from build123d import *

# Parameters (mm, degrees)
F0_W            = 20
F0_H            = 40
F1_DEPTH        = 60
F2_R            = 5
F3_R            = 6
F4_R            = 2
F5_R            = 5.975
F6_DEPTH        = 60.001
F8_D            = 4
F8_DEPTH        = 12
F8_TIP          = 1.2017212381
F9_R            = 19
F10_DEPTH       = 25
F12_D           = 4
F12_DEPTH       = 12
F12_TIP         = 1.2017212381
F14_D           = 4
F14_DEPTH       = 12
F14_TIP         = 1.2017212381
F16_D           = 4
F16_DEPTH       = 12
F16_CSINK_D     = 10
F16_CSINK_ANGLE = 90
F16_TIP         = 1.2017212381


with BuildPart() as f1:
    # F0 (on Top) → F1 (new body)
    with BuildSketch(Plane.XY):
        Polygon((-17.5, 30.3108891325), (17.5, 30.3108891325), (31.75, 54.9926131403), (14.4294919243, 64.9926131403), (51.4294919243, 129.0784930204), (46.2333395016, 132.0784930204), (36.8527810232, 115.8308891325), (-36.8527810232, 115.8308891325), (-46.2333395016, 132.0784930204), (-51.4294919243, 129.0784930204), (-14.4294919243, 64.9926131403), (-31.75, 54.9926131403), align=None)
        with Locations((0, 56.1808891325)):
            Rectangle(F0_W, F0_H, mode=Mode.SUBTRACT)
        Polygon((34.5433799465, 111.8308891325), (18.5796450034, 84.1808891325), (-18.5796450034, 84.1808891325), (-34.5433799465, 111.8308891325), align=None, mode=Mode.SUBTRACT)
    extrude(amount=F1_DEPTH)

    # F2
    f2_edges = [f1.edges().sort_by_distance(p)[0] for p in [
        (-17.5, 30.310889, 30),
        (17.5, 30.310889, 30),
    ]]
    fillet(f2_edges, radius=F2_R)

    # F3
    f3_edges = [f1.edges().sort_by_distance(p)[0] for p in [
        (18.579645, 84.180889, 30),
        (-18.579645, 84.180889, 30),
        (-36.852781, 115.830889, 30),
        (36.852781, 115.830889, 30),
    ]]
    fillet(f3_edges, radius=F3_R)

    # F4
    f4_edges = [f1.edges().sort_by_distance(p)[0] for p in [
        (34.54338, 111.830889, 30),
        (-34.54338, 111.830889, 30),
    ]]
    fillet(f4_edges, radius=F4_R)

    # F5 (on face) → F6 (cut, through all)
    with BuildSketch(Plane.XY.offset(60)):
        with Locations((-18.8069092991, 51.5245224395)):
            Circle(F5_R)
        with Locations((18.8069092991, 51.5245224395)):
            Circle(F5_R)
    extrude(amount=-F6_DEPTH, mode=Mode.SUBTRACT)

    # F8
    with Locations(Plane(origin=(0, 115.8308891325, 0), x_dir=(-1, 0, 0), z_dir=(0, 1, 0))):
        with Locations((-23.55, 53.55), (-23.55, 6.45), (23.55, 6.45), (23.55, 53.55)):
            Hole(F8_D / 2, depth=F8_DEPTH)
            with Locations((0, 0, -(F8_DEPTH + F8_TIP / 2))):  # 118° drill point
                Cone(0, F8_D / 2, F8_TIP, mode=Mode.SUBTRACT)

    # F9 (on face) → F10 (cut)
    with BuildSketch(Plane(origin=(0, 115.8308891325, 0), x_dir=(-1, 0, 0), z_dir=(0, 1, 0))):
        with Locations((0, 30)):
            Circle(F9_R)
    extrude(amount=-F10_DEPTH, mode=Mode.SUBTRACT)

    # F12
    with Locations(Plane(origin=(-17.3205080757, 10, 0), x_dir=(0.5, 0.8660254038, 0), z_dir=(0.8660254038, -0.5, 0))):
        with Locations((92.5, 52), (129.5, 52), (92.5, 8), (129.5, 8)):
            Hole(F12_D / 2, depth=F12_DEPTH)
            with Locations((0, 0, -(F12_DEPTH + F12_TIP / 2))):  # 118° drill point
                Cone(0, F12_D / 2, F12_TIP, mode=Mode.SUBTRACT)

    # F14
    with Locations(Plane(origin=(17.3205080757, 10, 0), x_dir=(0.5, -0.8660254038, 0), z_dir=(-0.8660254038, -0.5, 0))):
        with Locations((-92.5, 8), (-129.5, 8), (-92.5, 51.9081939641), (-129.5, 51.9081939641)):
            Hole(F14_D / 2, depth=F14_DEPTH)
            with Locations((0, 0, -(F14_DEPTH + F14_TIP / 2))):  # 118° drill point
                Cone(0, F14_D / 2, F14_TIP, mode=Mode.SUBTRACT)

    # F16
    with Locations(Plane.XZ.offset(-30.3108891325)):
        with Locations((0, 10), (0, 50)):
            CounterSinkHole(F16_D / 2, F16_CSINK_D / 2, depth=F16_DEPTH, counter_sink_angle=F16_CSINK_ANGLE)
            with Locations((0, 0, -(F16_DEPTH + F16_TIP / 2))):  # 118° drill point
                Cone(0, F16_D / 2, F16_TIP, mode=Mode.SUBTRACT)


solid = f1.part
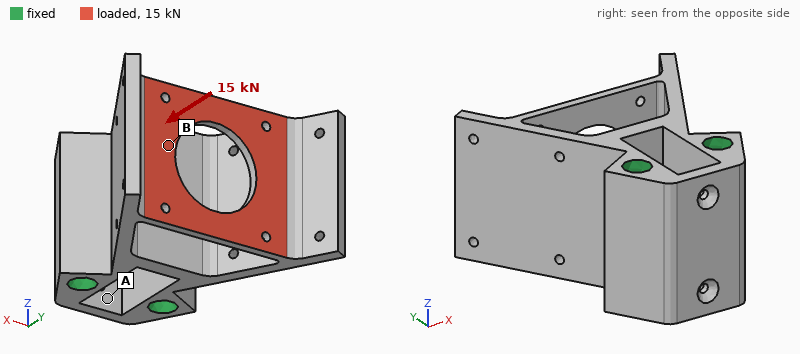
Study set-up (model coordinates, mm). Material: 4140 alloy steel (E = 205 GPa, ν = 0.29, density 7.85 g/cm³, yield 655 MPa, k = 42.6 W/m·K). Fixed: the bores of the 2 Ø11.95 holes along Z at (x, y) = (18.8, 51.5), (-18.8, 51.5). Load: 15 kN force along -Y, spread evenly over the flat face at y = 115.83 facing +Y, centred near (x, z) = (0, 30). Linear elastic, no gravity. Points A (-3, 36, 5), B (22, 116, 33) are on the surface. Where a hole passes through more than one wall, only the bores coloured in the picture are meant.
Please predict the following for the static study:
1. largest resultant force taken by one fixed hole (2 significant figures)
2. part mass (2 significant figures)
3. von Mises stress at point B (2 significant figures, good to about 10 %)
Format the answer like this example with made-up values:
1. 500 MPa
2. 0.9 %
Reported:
1. 9.0 kN
2. 1.1 kg
3. 100 MPa
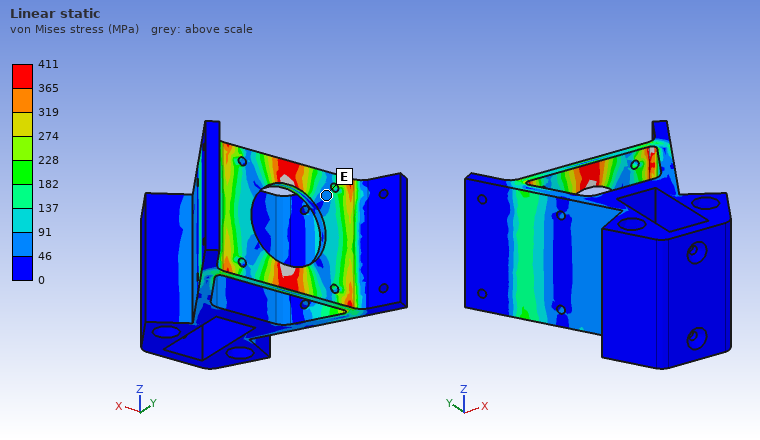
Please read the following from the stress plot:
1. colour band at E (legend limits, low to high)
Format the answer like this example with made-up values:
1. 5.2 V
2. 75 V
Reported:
1. 46 to 91 MPa
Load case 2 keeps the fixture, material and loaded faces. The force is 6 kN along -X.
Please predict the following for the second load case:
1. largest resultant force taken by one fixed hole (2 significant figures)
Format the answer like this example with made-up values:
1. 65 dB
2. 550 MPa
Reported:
1. 10 kN
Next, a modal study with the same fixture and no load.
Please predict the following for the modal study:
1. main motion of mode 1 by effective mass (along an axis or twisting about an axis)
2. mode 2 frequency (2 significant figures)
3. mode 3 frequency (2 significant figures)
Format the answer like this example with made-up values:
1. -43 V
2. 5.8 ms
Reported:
1. along X
2. 4000 Hz
3. 4200 Hz
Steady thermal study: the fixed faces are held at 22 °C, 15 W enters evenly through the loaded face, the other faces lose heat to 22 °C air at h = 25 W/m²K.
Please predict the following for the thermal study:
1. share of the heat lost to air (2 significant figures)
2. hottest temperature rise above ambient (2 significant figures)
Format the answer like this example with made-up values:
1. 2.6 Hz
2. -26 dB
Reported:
1. 52 %
2. 28 K
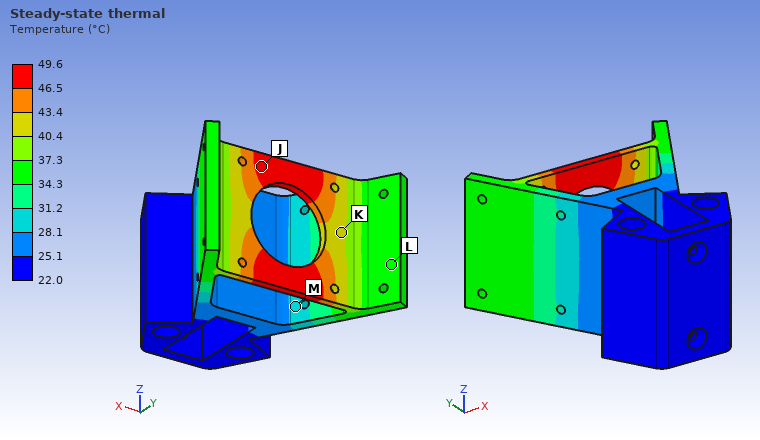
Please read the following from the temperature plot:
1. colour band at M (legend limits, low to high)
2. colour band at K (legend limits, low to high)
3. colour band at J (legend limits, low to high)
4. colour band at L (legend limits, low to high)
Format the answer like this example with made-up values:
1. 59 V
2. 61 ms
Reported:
1. 28.1 to 31.2 °C
2. 40.4 to 43.4 °C
3. 46.5 to 49.6 °C
4. 34.3 to 37.3 °C
